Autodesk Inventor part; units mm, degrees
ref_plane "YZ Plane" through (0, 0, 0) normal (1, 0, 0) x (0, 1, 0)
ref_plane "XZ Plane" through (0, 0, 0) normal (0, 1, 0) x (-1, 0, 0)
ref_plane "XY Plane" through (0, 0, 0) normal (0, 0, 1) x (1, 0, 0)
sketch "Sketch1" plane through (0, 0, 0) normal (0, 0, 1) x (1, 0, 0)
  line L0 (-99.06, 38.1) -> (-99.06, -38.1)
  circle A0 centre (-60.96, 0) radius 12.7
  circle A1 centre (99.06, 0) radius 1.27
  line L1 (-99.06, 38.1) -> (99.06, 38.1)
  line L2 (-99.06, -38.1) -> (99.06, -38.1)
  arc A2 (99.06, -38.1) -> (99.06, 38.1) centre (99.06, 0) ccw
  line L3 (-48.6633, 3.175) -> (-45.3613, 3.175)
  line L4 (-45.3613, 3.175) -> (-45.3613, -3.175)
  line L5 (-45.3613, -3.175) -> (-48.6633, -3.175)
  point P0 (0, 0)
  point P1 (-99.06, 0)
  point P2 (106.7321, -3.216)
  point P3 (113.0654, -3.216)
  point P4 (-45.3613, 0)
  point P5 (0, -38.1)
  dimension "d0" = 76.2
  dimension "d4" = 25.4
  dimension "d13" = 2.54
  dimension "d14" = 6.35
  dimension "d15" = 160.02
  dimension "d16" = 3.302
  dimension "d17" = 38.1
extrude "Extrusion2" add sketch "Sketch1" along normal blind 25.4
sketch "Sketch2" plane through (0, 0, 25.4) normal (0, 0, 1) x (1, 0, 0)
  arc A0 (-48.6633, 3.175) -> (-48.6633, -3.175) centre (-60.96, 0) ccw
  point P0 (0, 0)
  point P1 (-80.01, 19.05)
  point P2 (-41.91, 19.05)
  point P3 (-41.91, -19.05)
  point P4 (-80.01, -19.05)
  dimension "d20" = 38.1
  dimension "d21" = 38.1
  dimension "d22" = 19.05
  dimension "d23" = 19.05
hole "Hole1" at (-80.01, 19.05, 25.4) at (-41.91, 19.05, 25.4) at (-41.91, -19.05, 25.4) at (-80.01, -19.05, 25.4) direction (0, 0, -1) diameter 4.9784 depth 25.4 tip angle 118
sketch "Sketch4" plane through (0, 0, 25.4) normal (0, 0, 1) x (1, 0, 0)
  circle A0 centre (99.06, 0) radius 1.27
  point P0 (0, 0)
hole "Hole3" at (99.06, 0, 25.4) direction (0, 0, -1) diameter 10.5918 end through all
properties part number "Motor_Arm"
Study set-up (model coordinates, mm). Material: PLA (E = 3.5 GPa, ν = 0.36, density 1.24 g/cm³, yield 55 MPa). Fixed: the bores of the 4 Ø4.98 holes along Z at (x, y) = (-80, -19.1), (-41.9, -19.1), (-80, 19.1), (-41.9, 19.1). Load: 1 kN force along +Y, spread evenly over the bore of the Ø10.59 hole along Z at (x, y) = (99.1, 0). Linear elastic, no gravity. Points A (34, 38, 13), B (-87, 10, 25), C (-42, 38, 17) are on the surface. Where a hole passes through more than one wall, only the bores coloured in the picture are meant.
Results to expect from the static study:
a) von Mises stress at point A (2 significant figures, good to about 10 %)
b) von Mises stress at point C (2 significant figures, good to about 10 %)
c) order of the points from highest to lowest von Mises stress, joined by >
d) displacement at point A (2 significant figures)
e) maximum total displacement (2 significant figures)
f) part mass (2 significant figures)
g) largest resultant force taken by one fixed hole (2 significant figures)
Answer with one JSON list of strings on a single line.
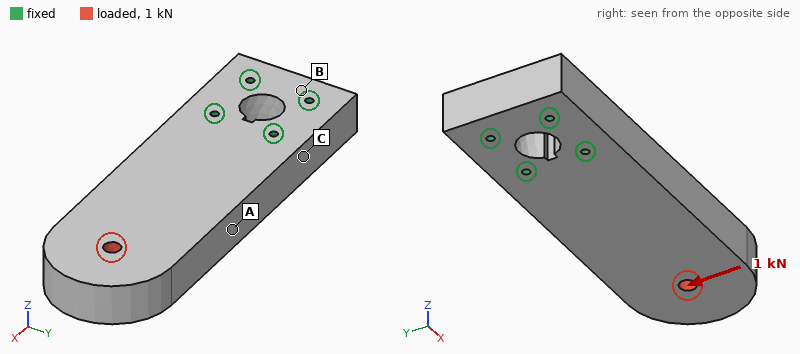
["2.6 MPa", "4.4 MPa", "C > A > B", "0.22 mm", "0.57 mm", "530 g", "2.4 kN"]
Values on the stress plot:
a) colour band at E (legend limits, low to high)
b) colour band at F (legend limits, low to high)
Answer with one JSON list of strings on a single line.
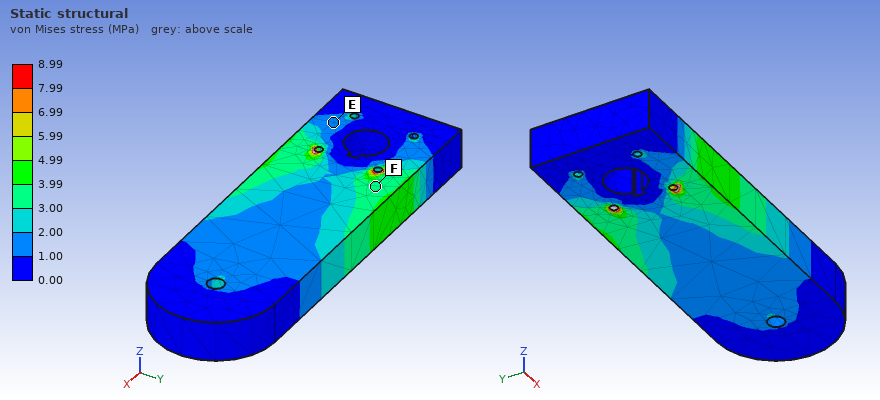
["1.00 to 2.00 MPa", "3.00 to 3.99 MPa"]
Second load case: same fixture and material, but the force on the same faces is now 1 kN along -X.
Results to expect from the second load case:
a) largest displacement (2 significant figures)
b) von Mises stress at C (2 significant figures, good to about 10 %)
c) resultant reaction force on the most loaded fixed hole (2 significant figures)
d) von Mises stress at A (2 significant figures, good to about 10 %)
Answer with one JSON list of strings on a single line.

["28 µm", "0.36 MPa", "430 N", "0.51 MPa"]
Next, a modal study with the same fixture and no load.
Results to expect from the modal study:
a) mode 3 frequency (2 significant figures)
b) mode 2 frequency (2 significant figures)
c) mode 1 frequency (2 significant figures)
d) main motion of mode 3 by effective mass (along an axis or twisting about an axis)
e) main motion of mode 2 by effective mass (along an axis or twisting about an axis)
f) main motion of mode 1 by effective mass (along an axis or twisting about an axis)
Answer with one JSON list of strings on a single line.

["920 Hz", "550 Hz", "220 Hz", "twisting about X", "along Y", "along Z"]
